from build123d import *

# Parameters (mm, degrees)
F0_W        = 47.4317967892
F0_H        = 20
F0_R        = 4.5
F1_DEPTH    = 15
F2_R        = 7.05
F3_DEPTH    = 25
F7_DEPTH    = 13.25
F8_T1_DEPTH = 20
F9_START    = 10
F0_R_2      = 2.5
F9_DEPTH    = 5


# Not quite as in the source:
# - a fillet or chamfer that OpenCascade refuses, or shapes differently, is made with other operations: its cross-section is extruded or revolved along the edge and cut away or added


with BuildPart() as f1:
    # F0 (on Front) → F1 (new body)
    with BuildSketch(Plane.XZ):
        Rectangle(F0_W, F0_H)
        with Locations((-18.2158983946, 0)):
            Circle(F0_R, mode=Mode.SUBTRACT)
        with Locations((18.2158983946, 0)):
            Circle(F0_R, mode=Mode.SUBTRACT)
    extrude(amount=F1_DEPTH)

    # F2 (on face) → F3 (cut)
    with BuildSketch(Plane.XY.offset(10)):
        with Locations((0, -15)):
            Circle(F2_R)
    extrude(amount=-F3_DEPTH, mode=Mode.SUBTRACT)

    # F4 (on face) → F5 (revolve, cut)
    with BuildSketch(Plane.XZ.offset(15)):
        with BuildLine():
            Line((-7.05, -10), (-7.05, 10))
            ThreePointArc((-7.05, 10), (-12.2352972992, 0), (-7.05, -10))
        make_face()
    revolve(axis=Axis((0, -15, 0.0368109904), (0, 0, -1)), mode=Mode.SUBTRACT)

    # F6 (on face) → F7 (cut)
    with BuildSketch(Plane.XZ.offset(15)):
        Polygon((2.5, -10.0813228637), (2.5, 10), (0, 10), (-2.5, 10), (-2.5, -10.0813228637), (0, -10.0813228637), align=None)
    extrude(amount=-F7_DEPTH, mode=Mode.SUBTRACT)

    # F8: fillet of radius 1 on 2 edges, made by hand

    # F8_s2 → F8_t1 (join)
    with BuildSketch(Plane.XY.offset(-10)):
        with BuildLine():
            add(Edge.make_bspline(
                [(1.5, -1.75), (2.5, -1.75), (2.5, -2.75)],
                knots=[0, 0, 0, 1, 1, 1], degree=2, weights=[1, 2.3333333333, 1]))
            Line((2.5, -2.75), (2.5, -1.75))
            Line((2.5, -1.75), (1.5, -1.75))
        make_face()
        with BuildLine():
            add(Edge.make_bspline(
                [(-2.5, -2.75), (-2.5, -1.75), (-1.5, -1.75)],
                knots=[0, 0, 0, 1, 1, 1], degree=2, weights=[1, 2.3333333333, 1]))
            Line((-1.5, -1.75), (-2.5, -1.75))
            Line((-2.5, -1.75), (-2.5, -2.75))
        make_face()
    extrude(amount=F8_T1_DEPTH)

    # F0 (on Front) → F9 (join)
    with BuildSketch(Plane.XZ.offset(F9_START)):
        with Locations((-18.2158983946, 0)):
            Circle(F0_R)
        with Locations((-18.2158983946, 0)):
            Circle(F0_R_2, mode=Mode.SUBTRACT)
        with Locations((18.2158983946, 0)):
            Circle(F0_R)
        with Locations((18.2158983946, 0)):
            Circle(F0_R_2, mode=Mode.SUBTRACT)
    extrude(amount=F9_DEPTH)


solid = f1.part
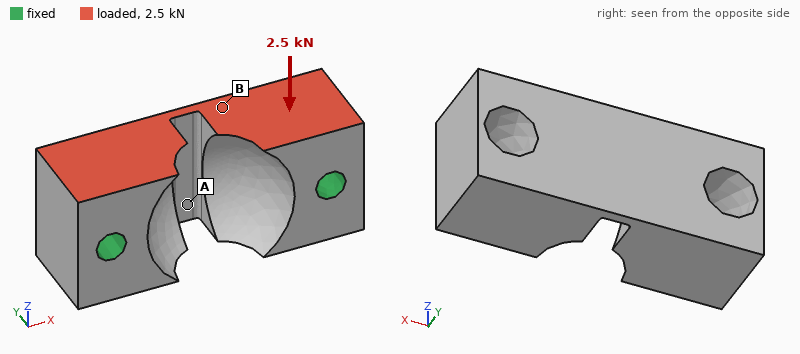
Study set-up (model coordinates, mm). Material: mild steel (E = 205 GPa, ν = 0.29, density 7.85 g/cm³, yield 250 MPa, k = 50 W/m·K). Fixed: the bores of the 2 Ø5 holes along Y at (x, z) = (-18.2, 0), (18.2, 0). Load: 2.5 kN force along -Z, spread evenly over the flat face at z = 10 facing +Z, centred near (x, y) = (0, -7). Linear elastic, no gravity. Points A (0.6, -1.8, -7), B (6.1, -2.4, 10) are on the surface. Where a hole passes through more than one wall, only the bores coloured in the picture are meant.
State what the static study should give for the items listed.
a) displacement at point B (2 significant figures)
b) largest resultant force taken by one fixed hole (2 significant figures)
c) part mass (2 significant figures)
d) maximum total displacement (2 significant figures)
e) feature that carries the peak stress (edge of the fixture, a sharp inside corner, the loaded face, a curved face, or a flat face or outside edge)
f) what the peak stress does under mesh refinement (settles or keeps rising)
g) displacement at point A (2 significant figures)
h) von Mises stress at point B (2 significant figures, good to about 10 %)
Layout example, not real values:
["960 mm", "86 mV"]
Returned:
["6.2 µm", "1.3 kN", "69 g", "7.3 µm", "edge of the fixture", "keeps rising", "6.0 µm", "9.8 MPa"]
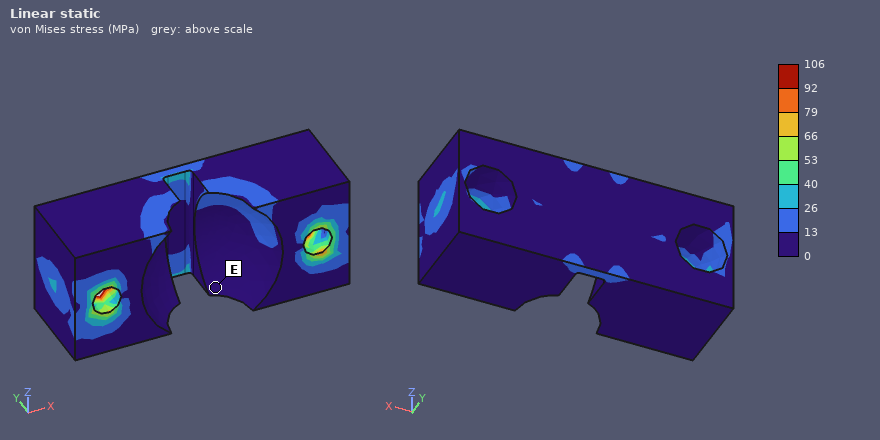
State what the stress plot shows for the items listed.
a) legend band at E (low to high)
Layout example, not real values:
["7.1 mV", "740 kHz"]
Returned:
["0 to 13 MPa"]
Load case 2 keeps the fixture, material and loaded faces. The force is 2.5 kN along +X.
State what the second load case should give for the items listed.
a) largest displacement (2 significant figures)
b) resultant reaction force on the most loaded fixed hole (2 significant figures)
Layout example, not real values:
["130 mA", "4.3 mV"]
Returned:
["6.6 µm", "1.3 kN"]
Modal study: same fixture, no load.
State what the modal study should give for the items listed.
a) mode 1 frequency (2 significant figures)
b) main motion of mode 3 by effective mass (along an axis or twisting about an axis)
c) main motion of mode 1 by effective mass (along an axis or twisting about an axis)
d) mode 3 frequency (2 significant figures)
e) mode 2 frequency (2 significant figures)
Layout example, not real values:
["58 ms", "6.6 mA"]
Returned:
["13 kHz", "along X", "along Z", "19 kHz", "18 kHz"]
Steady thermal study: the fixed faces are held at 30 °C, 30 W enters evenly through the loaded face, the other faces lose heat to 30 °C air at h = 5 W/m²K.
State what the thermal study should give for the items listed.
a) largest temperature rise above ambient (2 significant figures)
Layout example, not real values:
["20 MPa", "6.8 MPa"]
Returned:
["32 K"]
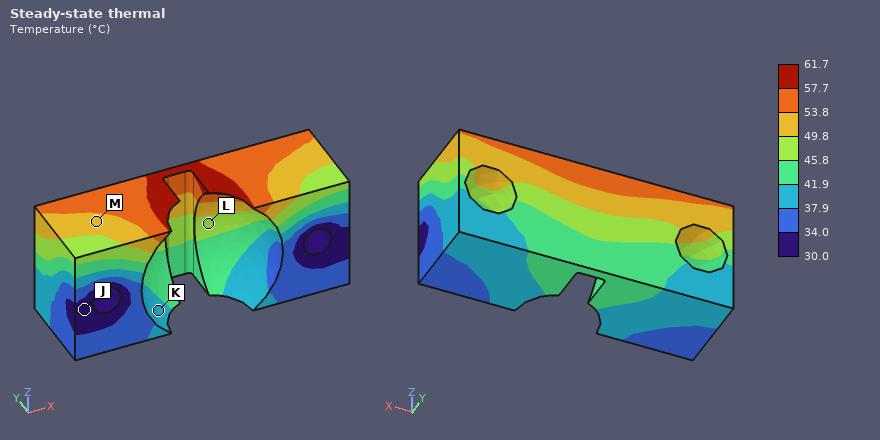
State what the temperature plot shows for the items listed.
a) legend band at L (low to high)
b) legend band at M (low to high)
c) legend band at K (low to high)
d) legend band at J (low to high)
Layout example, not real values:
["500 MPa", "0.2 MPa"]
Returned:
["45.8 to 49.8 °C", "49.8 to 53.8 °C", "37.9 to 41.9 °C", "30.0 to 34.0 °C"]
